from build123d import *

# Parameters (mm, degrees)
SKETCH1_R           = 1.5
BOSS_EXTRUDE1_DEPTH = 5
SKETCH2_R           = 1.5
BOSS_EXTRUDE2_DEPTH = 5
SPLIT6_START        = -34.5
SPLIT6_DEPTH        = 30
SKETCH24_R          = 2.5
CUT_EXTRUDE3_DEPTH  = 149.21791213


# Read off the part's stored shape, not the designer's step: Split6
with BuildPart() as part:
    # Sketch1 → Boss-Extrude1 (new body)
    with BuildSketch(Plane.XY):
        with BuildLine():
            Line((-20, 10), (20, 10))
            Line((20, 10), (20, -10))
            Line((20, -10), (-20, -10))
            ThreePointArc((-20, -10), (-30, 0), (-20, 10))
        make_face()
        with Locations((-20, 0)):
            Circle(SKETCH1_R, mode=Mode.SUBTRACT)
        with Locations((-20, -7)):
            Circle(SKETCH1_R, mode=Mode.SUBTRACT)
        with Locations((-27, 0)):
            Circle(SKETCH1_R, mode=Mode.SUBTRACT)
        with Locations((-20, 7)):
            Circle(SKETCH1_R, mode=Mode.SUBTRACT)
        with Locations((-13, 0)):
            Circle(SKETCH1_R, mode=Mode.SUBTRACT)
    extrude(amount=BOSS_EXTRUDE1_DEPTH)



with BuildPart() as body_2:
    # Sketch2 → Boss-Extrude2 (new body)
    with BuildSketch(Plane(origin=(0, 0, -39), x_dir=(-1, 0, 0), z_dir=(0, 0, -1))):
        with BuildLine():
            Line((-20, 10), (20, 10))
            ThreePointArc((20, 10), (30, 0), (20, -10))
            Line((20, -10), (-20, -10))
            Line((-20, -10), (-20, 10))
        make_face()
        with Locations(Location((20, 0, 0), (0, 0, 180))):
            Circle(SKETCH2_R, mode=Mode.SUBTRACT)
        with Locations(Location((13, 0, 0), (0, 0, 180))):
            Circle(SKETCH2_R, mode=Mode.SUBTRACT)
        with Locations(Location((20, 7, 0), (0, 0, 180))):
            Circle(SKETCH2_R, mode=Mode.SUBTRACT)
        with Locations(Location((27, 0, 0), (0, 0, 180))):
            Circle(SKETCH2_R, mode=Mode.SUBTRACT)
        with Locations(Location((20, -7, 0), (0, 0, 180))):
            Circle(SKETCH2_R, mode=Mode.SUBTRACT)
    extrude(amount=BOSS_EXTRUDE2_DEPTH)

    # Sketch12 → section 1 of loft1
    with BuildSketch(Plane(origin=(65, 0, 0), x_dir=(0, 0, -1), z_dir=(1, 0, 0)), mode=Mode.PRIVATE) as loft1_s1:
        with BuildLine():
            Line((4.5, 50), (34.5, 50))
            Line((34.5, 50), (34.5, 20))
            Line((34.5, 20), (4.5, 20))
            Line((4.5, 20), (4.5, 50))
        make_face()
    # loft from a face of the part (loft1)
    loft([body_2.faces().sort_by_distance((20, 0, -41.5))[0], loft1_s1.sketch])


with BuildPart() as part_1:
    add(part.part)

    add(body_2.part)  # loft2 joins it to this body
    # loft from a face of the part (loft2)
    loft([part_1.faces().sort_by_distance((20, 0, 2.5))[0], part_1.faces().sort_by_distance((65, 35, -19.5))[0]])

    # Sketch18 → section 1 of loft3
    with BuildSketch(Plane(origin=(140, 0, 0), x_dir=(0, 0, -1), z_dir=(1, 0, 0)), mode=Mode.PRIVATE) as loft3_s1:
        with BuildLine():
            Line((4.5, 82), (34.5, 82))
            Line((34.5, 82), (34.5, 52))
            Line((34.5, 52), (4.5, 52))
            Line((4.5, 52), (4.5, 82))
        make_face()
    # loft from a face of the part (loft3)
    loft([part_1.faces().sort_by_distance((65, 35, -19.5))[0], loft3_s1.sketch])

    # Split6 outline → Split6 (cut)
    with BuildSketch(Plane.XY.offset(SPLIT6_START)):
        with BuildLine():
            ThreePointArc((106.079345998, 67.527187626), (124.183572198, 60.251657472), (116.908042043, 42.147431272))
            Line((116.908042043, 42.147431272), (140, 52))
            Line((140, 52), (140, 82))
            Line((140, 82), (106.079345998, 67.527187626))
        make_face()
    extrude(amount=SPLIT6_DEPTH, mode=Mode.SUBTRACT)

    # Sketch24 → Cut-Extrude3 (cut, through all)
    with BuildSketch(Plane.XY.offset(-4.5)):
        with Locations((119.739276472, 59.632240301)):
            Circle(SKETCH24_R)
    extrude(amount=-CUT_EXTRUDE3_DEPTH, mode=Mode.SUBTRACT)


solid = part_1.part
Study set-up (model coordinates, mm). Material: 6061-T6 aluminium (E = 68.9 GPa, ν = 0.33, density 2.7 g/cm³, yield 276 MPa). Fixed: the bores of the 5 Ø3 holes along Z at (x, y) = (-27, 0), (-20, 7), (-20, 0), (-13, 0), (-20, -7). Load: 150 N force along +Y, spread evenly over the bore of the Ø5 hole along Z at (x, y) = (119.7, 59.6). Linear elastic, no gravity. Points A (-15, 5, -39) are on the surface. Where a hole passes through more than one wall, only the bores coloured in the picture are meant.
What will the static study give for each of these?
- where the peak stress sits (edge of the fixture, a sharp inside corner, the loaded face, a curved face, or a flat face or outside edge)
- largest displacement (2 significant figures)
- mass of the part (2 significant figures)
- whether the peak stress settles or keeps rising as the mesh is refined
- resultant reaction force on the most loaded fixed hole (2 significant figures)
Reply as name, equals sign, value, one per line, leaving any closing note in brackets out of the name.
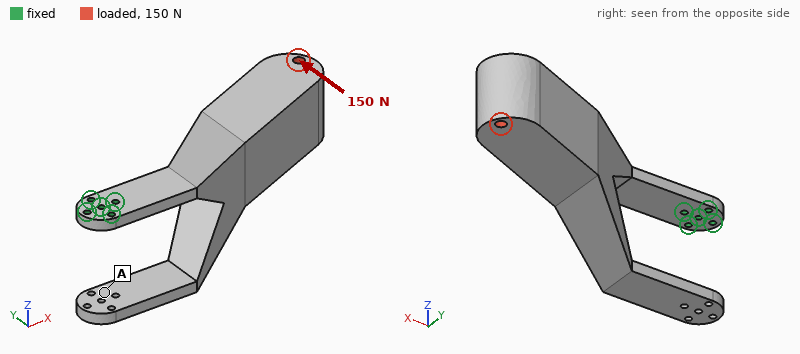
where the peak stress sits = edge of the fixture
largest displacement = 0.83 mm
mass of the part = 250 g
whether the peak stress settles or keeps rising as the mesh is refined = keeps rising
resultant reaction force on the most loaded fixed hole = 1.0 kN
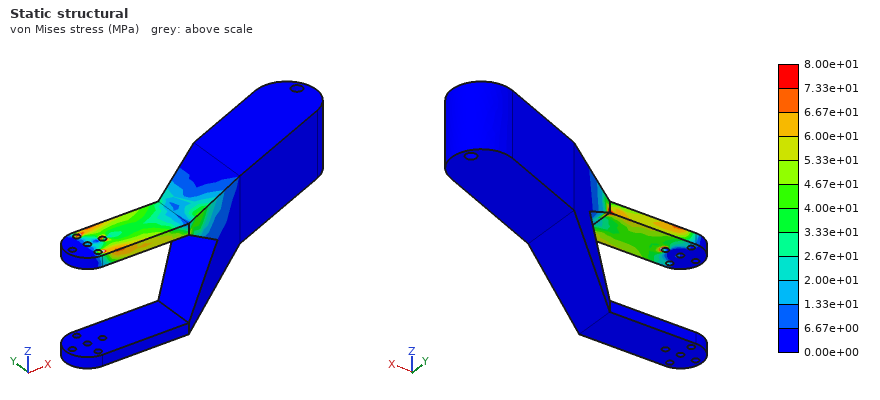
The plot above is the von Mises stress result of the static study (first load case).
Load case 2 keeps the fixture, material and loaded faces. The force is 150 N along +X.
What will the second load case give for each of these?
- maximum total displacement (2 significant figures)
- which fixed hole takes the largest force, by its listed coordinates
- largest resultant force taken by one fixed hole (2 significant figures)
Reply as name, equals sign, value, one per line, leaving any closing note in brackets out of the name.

maximum total displacement = 1.3 mm
which fixed hole takes the largest force, by its listed coordinates = (-20, 7)
largest resultant force taken by one fixed hole = 500 N
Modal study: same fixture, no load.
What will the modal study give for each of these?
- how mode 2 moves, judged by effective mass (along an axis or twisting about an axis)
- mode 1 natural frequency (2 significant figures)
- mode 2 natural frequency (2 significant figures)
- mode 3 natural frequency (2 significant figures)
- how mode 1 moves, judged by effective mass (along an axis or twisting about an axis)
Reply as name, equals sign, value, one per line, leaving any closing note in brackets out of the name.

how mode 2 moves, judged by effective mass = along Y
mode 1 natural frequency = 74 Hz
mode 2 natural frequency = 200 Hz
mode 3 natural frequency = 430 Hz
how mode 1 moves, judged by effective mass = along Z
